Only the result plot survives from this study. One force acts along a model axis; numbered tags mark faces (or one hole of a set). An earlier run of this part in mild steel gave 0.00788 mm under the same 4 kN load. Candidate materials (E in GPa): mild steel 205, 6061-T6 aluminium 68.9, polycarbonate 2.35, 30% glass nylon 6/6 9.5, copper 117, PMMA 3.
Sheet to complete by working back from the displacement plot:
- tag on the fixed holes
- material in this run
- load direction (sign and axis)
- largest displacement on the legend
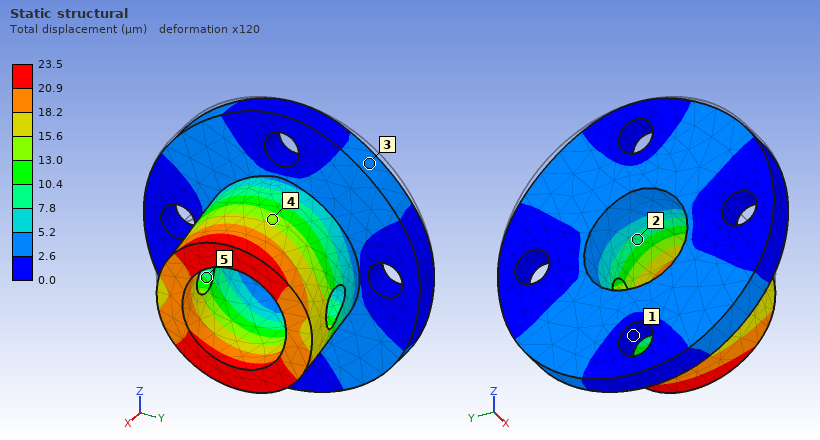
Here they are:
1
6061-T6 aluminium
-Z
23.5 µm
